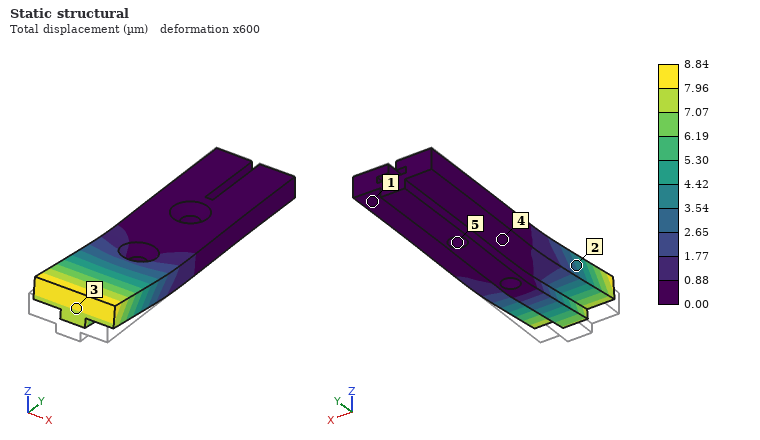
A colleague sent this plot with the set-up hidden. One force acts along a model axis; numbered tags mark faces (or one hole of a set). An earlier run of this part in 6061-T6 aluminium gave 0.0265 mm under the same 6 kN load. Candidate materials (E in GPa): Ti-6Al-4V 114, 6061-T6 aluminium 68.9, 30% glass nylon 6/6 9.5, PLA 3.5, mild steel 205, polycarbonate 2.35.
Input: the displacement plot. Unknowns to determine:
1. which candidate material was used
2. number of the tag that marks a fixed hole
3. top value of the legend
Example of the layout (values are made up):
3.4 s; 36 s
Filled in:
mild steel; 5; 8.84 µm
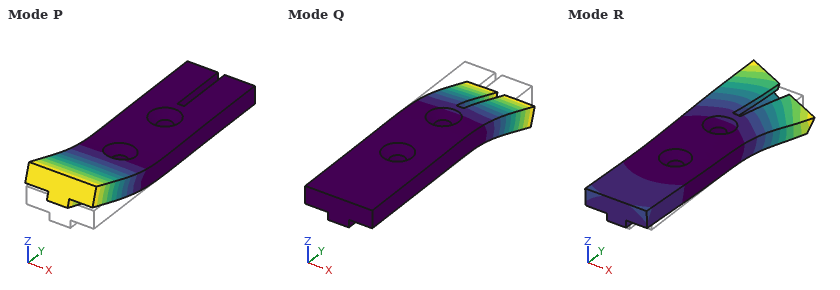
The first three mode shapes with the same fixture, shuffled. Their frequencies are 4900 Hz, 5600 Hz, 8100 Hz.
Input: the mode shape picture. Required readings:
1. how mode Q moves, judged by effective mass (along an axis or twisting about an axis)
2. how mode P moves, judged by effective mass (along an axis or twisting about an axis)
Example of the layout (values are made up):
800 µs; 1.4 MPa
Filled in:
along Z; along Z
